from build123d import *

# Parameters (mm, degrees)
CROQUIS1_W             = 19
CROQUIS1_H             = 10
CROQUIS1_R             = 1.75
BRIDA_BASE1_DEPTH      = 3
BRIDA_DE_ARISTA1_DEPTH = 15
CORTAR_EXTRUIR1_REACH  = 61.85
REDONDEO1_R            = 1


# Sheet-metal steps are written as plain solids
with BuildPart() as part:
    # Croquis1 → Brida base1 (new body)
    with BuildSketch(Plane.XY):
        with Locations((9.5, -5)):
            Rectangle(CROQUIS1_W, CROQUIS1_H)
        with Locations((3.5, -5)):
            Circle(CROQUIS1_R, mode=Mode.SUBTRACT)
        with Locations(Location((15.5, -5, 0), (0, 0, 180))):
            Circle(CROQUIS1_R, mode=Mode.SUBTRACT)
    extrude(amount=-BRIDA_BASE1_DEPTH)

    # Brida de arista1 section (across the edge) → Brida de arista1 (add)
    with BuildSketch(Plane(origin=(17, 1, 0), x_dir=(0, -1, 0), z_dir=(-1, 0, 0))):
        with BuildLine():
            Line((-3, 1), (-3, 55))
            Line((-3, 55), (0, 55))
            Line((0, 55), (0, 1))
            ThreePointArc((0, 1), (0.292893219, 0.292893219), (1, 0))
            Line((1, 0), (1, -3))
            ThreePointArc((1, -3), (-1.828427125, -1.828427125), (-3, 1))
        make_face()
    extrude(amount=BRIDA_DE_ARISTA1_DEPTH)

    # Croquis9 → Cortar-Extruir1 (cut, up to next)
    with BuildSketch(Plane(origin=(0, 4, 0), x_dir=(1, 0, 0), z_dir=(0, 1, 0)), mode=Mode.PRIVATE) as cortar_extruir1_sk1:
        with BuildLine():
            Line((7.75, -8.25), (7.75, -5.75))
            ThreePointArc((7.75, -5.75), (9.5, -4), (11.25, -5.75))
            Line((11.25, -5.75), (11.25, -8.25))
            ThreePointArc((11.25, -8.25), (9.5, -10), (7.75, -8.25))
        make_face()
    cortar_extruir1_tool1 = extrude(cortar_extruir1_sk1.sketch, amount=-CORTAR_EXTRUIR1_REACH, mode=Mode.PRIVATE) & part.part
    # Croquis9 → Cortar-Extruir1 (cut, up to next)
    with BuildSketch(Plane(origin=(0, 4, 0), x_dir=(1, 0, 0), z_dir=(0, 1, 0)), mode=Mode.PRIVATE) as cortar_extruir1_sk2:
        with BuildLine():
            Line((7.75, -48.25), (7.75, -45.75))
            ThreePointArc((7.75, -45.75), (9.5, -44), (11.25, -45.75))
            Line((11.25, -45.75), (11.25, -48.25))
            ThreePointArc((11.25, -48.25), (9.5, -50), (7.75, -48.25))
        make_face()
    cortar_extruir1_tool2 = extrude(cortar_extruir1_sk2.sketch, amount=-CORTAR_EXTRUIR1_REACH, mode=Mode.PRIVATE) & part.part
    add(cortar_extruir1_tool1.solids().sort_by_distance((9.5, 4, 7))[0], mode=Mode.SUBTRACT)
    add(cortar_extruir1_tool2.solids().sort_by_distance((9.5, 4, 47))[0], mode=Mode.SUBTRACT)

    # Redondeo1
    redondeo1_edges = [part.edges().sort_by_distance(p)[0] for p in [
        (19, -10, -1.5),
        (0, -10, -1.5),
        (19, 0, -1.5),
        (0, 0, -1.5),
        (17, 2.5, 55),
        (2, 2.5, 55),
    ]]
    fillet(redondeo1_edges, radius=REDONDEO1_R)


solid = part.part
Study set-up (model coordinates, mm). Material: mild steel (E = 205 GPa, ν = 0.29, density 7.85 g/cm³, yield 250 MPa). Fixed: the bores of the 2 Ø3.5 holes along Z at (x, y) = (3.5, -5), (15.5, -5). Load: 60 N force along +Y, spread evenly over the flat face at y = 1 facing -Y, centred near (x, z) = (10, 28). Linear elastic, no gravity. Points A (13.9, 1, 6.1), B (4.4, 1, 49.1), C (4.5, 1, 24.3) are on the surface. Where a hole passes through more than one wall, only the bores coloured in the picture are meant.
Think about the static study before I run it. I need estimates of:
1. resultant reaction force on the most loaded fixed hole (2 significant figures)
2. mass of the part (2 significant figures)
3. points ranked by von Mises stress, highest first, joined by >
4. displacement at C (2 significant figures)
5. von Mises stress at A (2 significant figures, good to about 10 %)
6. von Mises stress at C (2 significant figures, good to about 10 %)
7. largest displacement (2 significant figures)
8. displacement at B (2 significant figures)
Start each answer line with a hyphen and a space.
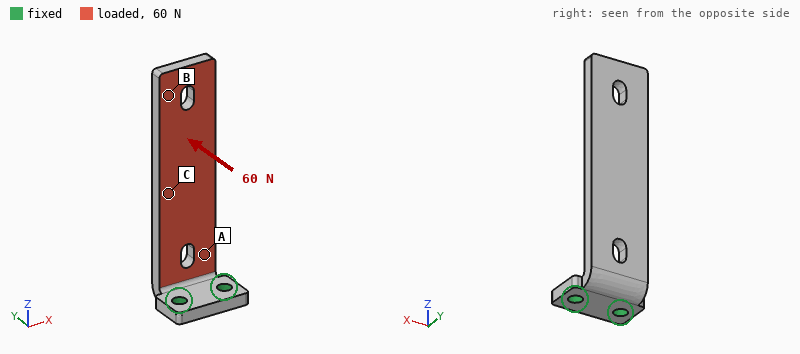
- 38 N
- 24 g
- A > C > B
- 0.10 mm
- 74 MPa
- 23 MPa
- 0.29 mm
- 0.26 mm
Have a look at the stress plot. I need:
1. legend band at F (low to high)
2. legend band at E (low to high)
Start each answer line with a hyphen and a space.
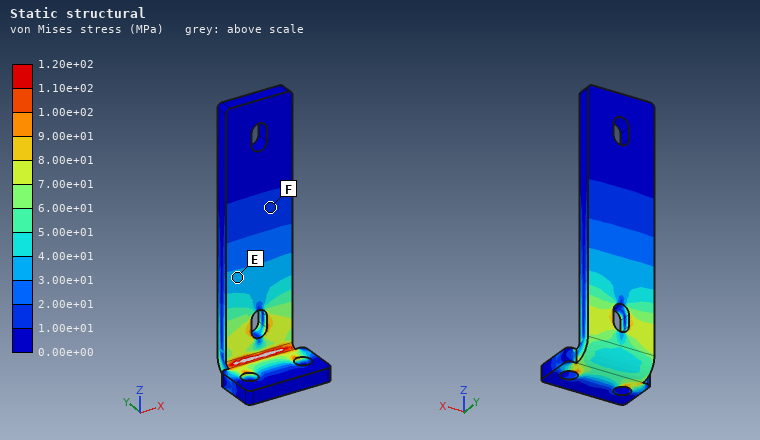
- 1.00e+01 to 2.00e+01 MPa
- 3.00e+01 to 4.00e+01 MPa
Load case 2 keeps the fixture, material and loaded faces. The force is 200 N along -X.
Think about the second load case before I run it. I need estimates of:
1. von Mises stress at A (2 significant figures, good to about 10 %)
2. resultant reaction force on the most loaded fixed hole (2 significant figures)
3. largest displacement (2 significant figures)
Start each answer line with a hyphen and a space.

- 57 MPa
- 490 N
- 0.10 mm
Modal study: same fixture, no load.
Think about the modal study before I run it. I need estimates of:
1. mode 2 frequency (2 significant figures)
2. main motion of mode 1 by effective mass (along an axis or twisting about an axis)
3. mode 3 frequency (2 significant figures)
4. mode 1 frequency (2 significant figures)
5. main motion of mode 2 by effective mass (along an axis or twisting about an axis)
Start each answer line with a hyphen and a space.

- 2100 Hz
- along Y
- 4300 Hz
- 660 Hz
- along X
